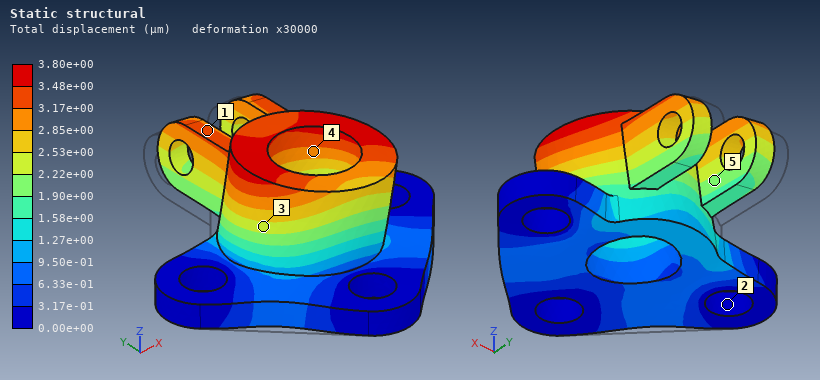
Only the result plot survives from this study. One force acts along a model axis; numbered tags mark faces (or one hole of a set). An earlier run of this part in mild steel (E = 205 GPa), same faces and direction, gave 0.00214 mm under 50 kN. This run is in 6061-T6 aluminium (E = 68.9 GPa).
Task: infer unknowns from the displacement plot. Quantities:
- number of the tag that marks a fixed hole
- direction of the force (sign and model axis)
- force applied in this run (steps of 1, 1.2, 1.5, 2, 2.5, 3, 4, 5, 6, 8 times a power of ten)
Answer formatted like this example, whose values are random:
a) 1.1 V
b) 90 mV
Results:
a) 2
b) +X
c) 30 kN
